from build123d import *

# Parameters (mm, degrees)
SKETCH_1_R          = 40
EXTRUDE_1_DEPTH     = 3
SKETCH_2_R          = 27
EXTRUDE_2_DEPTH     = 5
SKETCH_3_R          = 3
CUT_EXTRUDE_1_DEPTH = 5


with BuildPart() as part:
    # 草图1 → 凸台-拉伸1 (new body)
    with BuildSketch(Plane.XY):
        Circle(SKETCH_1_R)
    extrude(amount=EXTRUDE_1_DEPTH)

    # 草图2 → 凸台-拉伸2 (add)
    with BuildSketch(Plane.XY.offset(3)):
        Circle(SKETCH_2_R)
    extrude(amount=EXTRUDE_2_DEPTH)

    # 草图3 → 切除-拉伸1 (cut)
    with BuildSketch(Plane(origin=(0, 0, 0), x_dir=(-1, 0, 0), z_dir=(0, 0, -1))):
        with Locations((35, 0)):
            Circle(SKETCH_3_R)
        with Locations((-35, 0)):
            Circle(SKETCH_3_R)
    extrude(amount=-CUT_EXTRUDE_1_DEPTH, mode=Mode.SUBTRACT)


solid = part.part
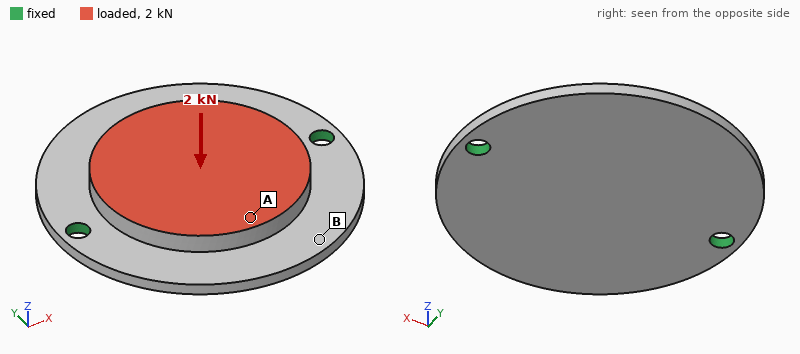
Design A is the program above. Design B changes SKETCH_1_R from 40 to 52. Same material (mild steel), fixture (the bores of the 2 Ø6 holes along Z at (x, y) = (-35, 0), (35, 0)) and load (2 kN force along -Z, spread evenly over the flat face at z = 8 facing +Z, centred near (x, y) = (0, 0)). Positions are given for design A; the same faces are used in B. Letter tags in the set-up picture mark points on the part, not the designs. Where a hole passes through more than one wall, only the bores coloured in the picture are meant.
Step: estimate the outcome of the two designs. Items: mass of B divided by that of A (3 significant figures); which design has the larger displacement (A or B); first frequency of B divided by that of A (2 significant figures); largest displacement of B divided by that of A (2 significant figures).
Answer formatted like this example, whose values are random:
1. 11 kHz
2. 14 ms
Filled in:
1. 1.39
2. B
3. 0.73
4. 1.1
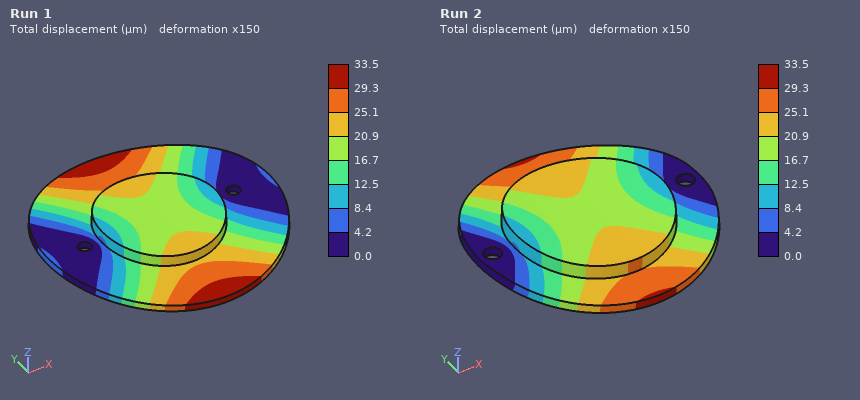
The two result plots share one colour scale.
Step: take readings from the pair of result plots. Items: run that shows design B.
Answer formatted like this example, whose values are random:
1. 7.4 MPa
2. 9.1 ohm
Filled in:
1. Run 1
